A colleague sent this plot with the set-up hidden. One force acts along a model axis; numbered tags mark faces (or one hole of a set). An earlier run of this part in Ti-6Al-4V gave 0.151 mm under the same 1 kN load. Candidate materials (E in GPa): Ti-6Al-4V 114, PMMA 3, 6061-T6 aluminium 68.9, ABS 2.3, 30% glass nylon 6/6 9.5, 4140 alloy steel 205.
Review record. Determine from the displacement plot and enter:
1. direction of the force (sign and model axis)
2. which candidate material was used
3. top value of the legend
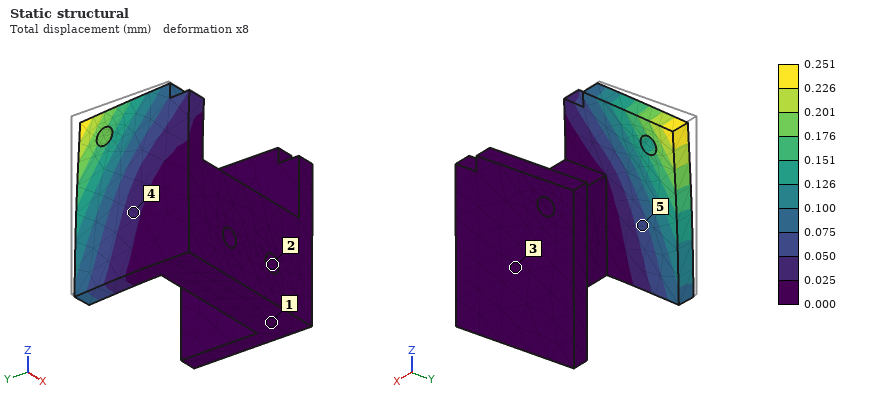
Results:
+X
6061-T6 aluminium
0.251 mm
